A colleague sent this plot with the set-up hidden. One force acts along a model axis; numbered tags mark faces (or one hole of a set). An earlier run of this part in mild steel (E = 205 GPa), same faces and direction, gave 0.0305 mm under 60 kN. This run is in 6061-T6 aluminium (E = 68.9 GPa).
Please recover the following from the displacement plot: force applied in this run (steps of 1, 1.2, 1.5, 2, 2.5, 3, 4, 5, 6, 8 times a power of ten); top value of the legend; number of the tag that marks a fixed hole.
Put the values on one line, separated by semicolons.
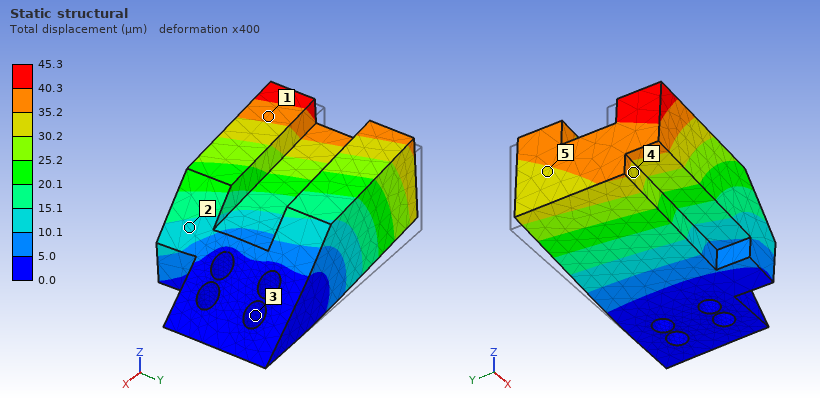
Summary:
30 kN; 45.3 µm; 3
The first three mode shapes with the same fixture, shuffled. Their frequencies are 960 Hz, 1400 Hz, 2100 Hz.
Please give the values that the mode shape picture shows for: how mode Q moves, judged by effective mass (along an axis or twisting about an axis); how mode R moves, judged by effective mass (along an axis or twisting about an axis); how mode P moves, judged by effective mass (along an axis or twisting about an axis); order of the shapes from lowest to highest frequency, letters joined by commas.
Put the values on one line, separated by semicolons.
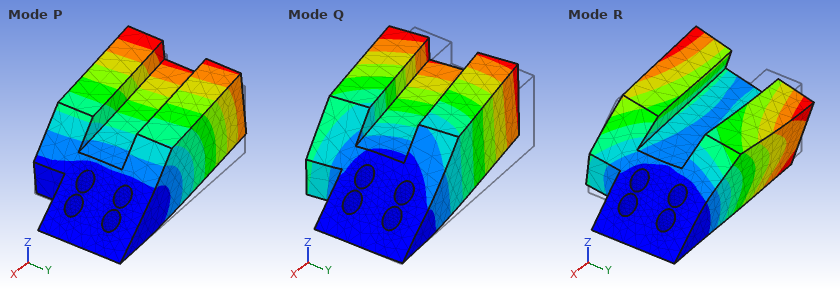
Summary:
along Y; twisting about X; along Z; P, Q, R
